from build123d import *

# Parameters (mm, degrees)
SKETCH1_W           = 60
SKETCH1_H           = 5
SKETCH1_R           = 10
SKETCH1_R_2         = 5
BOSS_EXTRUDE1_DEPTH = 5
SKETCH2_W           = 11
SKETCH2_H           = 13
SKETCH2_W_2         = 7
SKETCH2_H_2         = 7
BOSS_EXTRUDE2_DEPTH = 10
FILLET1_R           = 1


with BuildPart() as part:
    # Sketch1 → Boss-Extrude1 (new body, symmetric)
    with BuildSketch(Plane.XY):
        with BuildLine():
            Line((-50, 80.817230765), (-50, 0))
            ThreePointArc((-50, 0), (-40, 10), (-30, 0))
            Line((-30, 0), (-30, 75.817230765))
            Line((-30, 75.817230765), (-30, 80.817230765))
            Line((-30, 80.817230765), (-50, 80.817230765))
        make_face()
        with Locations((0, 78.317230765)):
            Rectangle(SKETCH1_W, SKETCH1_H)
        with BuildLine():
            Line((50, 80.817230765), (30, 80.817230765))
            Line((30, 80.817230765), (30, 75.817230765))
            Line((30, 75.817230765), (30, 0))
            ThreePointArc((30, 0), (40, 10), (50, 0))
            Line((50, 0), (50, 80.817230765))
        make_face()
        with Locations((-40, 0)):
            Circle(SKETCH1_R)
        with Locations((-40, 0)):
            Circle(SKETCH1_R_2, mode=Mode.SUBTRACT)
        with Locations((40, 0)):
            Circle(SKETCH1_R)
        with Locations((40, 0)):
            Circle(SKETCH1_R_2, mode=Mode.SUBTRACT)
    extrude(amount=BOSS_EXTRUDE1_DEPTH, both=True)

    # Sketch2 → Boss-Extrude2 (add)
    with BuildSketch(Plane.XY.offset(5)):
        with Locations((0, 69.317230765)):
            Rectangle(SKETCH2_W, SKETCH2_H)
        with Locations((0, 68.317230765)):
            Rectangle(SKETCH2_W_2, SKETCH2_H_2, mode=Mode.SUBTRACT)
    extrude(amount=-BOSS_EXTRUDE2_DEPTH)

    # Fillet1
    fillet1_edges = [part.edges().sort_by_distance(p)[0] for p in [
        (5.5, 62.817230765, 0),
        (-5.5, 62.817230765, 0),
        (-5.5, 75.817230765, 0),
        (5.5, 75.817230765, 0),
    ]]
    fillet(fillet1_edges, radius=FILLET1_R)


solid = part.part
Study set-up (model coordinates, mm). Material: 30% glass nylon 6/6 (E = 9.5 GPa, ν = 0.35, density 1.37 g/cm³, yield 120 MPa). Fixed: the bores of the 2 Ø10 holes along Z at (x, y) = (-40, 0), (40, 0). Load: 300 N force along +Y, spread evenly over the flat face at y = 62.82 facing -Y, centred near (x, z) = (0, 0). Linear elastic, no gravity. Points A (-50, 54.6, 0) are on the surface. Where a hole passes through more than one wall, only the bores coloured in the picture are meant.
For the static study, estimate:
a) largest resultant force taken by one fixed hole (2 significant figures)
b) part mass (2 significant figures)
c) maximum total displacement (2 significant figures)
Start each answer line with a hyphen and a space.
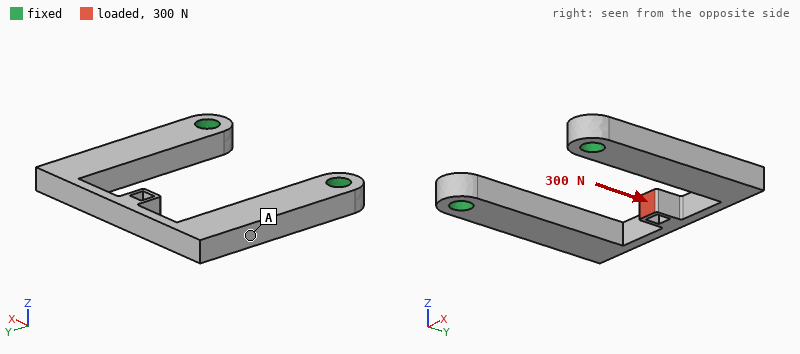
- 160 N
- 52 g
- 0.39 mm
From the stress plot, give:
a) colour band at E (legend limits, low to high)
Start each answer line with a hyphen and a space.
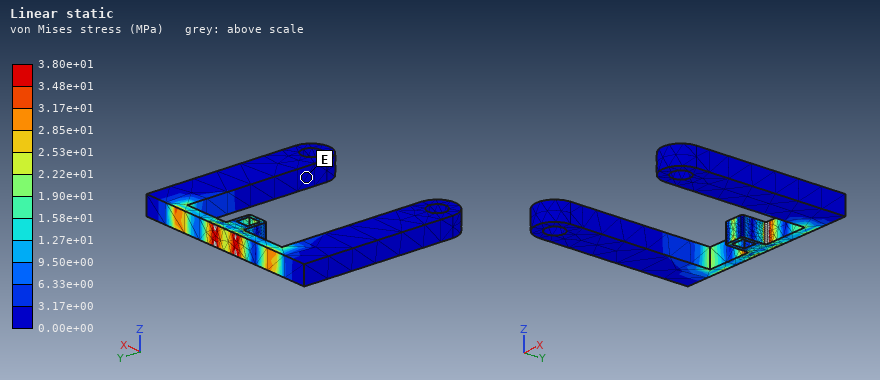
- 0.00e+00 to 3.17e+00 MPa
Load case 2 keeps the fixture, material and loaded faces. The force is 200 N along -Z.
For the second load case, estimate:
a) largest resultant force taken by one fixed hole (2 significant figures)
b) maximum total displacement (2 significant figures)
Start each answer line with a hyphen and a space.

- 100 N
- 1.4 mm
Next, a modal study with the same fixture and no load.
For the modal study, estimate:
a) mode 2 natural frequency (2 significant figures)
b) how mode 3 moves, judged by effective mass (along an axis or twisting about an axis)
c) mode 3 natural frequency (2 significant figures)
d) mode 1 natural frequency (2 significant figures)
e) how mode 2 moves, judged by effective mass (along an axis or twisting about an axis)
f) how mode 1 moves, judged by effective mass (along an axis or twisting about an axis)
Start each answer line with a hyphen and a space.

- 920 Hz
- along X
- 1000 Hz
- 580 Hz
- twisting about Y
- along Z
